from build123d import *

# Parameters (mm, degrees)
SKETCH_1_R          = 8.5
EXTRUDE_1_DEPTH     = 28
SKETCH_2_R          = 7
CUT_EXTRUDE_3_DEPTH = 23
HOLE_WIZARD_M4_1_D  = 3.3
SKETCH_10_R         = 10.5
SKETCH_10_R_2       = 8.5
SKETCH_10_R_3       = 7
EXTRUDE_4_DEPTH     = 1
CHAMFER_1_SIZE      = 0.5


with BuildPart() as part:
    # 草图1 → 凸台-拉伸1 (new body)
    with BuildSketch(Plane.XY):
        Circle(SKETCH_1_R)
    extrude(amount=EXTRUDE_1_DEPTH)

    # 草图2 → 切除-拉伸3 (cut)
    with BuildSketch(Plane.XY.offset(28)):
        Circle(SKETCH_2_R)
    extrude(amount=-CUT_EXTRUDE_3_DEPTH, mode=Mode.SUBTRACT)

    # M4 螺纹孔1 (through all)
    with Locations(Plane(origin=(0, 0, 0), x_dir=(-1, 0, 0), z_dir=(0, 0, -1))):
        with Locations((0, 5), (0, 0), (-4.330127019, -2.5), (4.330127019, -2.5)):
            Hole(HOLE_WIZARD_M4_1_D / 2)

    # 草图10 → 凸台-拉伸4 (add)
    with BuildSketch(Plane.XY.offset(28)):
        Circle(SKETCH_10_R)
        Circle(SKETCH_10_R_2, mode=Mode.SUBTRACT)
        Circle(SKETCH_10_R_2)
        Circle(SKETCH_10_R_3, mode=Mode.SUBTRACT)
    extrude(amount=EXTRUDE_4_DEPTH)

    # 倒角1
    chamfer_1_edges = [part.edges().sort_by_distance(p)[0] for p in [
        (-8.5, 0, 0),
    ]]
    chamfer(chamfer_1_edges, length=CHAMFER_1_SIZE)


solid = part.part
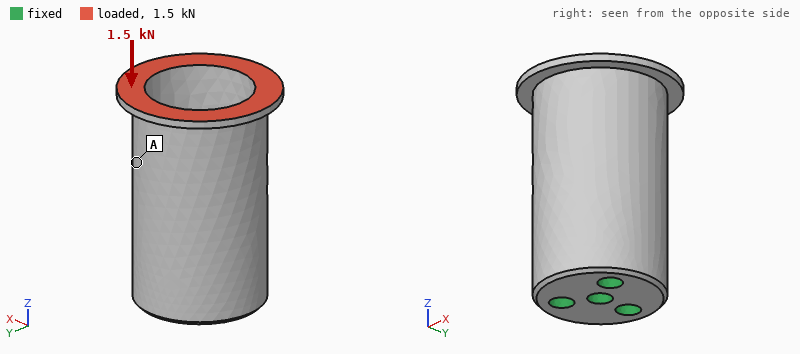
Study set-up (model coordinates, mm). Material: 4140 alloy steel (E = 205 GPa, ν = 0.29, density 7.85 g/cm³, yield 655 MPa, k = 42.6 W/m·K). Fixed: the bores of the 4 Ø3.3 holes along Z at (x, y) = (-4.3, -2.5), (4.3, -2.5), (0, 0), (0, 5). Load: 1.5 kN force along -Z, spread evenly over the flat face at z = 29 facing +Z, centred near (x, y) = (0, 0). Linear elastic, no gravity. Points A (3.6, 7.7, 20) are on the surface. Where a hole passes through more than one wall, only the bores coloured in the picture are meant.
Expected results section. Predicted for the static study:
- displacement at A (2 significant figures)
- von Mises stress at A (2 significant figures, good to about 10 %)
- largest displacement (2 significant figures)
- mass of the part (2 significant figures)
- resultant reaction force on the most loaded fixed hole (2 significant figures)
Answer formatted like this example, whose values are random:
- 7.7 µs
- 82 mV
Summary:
- 2.0 µm
- 18 MPa
- 6.7 µm
- 22 g
- 490 N
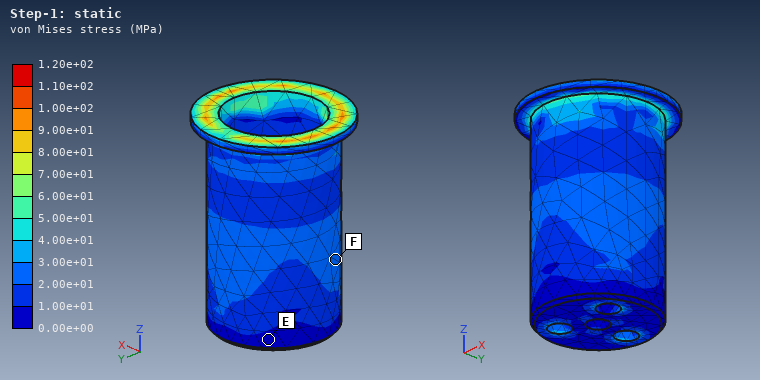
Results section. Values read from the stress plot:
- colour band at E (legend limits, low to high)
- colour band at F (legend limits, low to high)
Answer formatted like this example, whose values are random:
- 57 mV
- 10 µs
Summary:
- 0.00e+00 to 1.00e+01 MPa
- 2.00e+01 to 3.00e+01 MPa
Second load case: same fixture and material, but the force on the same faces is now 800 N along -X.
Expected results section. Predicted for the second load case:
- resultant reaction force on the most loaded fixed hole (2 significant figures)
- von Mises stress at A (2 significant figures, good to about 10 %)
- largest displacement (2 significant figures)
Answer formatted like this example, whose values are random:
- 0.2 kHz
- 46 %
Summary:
- 1.3 kN
- 33 MPa
- 25 µm
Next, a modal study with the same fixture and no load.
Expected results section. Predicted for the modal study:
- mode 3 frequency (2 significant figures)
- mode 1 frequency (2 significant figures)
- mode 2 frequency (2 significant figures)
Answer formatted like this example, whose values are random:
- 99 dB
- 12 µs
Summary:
- 21 kHz
- 13 kHz
- 13 kHz
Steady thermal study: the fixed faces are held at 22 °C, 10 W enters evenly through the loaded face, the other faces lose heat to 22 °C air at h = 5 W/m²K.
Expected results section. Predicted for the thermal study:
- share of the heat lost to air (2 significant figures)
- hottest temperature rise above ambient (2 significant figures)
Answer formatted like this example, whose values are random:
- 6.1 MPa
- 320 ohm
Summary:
- 5.6 %
- 82 K
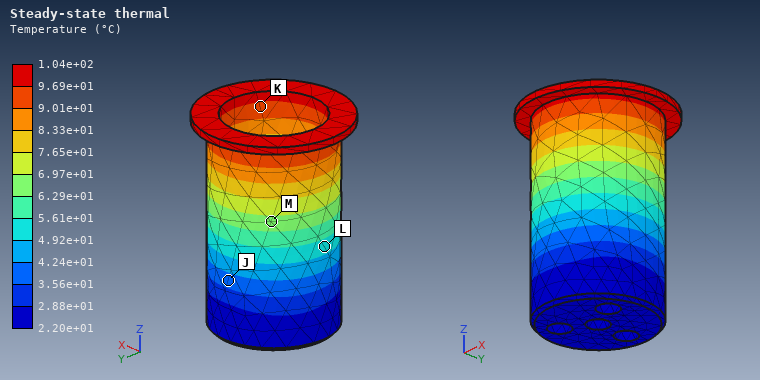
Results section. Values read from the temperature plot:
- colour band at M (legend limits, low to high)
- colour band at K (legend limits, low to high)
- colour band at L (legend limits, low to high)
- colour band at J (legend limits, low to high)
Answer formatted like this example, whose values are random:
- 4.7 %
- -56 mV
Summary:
- 6.29e+01 to 6.97e+01 °C
- 9.01e+01 to 9.69e+01 °C
- 4.92e+01 to 5.61e+01 °C
- 3.56e+01 to 4.24e+01 °C
